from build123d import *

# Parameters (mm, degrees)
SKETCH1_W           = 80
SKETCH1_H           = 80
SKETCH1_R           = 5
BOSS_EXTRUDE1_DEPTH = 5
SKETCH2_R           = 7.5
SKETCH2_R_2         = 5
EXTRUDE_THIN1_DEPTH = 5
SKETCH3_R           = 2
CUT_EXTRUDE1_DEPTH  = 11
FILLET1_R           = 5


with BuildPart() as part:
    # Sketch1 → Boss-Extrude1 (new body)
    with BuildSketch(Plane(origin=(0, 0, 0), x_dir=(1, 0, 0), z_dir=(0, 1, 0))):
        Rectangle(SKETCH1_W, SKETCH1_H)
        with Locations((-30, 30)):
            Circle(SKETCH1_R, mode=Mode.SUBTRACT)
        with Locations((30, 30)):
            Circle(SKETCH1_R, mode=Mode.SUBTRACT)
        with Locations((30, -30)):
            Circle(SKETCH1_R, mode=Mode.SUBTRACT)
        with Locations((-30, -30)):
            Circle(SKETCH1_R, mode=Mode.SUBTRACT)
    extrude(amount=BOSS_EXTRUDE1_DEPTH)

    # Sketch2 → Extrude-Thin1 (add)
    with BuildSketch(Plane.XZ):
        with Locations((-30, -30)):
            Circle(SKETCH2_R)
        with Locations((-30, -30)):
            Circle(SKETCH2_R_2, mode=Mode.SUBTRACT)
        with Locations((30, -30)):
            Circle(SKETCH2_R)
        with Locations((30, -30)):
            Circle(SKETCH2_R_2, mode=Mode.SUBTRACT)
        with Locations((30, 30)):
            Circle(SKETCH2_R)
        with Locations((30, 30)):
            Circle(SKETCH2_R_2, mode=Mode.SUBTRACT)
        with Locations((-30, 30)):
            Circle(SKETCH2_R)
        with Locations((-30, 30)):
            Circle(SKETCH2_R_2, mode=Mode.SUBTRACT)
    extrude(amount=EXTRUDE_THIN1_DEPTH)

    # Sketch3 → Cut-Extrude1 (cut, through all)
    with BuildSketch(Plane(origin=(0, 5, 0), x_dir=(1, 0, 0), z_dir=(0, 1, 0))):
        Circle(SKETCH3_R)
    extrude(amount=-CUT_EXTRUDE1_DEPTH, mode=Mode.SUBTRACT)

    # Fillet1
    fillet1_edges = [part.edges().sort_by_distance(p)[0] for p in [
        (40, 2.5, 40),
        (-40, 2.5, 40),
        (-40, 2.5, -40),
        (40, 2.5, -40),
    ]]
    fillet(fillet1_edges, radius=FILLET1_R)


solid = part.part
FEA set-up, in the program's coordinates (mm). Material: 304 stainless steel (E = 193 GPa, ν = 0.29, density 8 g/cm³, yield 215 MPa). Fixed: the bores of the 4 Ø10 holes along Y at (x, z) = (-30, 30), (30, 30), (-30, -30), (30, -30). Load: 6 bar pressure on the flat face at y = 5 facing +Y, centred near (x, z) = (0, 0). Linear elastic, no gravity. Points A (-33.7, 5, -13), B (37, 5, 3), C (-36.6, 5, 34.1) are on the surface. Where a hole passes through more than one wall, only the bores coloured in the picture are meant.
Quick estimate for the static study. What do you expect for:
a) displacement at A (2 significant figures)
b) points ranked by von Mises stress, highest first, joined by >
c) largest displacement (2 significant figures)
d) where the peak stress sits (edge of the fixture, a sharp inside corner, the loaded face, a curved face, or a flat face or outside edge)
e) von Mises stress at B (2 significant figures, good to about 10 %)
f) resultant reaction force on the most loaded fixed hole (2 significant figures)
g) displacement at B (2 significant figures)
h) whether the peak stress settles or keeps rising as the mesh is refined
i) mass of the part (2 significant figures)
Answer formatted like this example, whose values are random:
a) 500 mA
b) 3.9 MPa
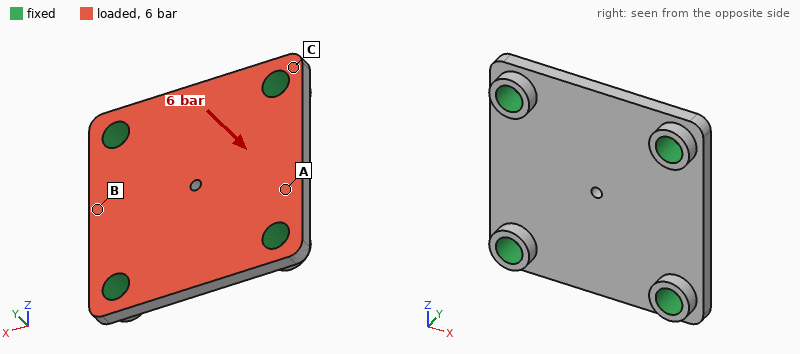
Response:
a) 3.8 µm
b) B > A > C
c) 16 µm
d) edge of the fixture
e) 17 MPa
f) 920 N
g) 5.8 µm
h) keeps rising
i) 260 g
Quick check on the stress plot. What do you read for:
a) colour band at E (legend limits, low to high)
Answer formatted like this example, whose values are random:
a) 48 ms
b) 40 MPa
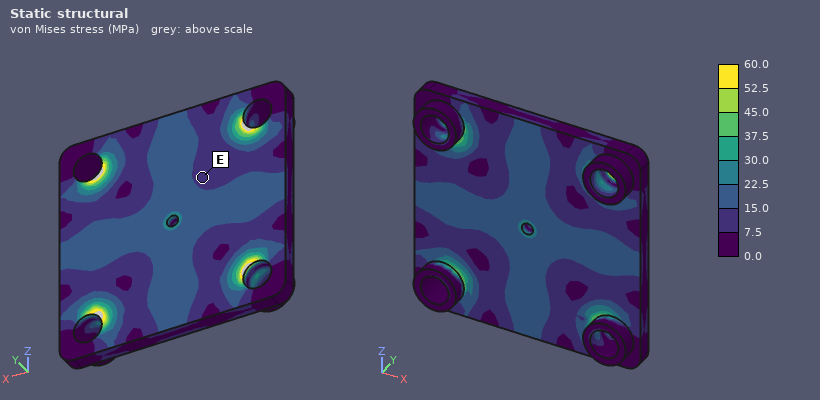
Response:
a) 7.5 to 15.0 MPa
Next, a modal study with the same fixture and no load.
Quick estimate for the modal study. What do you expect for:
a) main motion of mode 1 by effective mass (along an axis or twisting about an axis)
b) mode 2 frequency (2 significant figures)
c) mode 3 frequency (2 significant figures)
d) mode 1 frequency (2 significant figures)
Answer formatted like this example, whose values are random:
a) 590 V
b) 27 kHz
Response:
a) along Y
b) 9700 Hz
c) 9700 Hz
d) 6100 Hz
